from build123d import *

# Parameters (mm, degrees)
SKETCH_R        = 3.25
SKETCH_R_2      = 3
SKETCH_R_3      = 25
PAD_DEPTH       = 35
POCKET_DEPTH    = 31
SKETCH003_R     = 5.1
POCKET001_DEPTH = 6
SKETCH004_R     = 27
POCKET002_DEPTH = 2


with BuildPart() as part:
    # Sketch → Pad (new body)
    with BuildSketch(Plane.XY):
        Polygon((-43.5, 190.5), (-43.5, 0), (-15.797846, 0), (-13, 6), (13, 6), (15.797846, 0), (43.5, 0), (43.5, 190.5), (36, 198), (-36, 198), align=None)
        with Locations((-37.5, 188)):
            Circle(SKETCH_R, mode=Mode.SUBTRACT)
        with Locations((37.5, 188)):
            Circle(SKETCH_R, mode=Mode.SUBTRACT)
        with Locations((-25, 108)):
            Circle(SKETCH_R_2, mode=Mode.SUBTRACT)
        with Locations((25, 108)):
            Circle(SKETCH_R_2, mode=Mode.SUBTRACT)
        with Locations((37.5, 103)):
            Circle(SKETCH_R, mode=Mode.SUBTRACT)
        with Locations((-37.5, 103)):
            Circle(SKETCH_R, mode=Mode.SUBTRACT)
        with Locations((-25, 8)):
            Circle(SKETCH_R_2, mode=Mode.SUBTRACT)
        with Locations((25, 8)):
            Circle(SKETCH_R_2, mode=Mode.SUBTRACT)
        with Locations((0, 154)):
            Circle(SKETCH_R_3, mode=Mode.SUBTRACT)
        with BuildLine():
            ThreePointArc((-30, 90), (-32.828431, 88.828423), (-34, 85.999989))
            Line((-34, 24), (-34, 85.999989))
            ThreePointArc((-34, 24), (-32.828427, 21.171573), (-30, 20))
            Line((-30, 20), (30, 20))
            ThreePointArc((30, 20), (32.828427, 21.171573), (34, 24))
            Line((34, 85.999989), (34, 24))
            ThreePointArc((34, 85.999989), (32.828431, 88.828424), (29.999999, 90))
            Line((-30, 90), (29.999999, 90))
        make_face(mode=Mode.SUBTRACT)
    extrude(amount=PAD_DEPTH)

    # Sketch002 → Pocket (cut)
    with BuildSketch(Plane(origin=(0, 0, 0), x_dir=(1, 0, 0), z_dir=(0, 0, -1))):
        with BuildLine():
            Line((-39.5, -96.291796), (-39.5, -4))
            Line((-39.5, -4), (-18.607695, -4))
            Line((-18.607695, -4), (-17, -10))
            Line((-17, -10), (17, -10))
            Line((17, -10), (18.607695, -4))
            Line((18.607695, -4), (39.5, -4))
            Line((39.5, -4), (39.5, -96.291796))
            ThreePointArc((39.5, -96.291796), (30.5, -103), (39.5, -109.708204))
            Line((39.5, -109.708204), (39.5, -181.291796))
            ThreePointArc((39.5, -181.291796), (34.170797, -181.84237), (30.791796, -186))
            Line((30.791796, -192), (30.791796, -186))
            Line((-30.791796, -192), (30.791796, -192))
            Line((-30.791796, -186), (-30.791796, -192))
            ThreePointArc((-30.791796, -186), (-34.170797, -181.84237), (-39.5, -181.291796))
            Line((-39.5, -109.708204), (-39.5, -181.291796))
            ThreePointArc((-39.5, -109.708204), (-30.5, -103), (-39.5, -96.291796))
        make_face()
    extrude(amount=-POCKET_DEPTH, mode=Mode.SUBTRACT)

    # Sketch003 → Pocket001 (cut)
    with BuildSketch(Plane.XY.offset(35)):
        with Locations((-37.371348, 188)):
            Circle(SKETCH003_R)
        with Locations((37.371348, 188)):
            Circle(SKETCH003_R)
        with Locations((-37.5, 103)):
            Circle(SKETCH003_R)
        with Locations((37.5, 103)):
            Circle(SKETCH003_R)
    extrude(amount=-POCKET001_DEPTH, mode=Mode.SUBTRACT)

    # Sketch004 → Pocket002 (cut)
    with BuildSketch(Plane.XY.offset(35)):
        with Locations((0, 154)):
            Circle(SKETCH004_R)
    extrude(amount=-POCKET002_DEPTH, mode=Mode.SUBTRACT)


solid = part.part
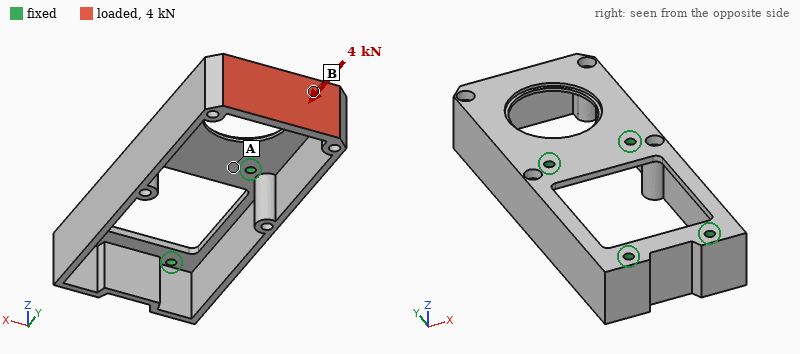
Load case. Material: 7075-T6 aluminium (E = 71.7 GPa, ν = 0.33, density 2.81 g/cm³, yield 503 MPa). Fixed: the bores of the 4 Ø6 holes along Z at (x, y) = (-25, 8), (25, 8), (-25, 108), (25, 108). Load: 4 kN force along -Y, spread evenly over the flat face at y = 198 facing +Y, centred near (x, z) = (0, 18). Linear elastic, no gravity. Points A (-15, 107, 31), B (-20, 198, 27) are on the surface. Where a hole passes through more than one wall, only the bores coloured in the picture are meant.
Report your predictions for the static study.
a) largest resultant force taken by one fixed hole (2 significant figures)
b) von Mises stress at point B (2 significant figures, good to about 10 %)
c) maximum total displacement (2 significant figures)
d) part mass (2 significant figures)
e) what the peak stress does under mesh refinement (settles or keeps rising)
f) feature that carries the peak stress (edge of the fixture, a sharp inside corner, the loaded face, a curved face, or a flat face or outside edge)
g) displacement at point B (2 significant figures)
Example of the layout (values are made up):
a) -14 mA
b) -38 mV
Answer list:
a) 1.3 kN
b) 32 MPa
c) 0.24 mm
d) 330 g
e) keeps rising
f) edge of the fixture
g) 0.14 mm
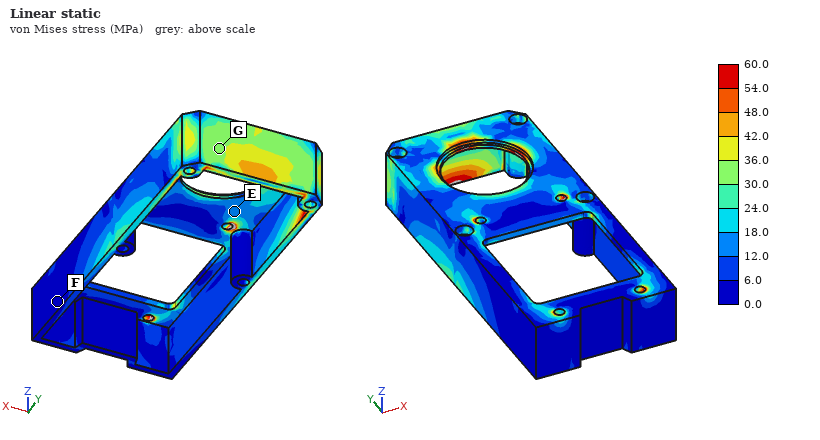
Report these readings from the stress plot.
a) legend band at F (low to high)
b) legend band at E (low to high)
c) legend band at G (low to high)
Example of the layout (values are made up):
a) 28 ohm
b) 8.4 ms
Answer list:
a) 0.0 to 6.0 MPa
b) 12.0 to 18.0 MPa
c) 30.0 to 36.0 MPa
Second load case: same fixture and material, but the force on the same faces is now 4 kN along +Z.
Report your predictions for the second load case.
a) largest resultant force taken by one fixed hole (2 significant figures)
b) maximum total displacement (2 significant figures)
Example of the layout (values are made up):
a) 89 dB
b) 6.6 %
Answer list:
a) 4.4 kN
b) 1.2 mm
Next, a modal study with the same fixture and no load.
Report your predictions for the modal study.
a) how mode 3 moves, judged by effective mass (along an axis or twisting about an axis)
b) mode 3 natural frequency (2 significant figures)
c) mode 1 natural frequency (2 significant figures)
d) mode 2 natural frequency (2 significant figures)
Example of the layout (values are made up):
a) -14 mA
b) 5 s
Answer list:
a) twisting about Z
b) 1900 Hz
c) 960 Hz
d) 990 Hz
